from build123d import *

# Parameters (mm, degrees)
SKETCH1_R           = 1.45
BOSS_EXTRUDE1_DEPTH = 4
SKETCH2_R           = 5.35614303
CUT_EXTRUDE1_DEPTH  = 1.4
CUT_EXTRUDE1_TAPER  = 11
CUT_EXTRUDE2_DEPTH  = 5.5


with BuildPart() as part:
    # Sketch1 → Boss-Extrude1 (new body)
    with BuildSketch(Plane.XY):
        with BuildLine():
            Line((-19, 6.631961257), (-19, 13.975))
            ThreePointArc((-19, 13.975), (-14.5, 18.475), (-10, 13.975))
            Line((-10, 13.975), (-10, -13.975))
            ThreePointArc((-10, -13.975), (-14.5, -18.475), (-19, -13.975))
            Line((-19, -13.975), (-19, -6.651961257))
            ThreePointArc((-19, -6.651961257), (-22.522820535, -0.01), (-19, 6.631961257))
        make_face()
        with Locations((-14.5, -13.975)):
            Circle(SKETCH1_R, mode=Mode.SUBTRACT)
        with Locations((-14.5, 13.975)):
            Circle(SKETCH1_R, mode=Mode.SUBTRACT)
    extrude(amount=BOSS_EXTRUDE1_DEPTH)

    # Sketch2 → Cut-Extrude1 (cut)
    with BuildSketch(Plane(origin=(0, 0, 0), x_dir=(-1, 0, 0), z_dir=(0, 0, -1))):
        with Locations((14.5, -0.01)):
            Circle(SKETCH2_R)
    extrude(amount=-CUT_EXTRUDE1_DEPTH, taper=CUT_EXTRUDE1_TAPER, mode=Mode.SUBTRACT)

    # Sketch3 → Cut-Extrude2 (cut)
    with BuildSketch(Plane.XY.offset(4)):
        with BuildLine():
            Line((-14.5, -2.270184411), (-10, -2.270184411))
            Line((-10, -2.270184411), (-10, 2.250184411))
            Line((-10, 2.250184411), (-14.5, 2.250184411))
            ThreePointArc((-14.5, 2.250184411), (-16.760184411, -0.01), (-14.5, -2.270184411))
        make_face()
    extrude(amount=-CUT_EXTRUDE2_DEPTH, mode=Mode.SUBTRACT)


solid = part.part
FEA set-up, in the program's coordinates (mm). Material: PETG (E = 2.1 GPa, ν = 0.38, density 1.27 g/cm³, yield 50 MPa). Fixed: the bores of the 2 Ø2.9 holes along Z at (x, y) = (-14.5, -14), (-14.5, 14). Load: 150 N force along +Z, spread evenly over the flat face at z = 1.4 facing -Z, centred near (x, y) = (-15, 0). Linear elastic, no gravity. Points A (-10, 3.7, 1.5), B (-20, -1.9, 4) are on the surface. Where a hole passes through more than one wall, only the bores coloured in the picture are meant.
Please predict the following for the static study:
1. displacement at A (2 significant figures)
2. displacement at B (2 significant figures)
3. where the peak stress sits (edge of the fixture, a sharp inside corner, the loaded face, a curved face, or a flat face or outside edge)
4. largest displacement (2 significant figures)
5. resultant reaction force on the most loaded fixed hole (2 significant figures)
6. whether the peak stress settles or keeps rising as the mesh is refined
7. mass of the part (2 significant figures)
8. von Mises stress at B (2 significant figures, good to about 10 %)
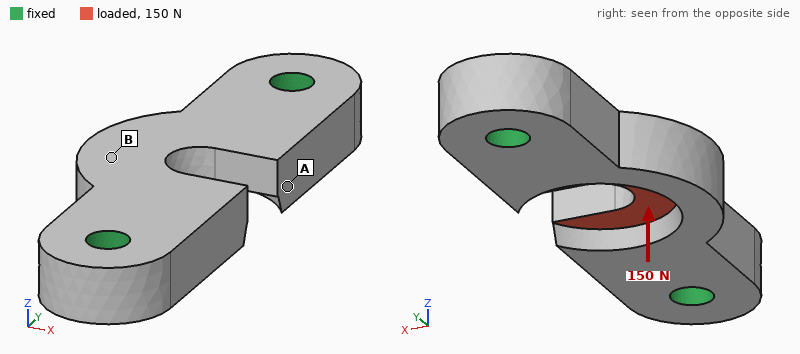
0.19 mm
0.24 mm
edge of the fixture
0.26 mm
78 N
keeps rising
1.5 g
15 MPa
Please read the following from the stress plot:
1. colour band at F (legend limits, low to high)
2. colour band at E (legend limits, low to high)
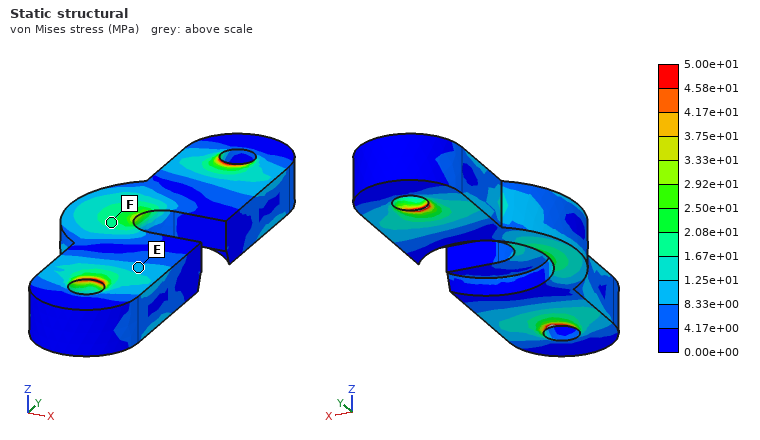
1.67e+01 to 2.08e+01 MPa
8.33e+00 to 1.25e+01 MPa
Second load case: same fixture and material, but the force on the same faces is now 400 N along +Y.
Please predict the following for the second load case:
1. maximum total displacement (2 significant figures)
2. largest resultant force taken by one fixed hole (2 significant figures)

59 µm
200 N
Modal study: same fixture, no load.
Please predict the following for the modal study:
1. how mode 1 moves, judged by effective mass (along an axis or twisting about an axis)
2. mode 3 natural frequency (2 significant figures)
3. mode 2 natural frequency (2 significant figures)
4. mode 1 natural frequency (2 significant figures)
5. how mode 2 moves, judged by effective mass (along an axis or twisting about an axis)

along Z
9200 Hz
8700 Hz
5400 Hz
along X
